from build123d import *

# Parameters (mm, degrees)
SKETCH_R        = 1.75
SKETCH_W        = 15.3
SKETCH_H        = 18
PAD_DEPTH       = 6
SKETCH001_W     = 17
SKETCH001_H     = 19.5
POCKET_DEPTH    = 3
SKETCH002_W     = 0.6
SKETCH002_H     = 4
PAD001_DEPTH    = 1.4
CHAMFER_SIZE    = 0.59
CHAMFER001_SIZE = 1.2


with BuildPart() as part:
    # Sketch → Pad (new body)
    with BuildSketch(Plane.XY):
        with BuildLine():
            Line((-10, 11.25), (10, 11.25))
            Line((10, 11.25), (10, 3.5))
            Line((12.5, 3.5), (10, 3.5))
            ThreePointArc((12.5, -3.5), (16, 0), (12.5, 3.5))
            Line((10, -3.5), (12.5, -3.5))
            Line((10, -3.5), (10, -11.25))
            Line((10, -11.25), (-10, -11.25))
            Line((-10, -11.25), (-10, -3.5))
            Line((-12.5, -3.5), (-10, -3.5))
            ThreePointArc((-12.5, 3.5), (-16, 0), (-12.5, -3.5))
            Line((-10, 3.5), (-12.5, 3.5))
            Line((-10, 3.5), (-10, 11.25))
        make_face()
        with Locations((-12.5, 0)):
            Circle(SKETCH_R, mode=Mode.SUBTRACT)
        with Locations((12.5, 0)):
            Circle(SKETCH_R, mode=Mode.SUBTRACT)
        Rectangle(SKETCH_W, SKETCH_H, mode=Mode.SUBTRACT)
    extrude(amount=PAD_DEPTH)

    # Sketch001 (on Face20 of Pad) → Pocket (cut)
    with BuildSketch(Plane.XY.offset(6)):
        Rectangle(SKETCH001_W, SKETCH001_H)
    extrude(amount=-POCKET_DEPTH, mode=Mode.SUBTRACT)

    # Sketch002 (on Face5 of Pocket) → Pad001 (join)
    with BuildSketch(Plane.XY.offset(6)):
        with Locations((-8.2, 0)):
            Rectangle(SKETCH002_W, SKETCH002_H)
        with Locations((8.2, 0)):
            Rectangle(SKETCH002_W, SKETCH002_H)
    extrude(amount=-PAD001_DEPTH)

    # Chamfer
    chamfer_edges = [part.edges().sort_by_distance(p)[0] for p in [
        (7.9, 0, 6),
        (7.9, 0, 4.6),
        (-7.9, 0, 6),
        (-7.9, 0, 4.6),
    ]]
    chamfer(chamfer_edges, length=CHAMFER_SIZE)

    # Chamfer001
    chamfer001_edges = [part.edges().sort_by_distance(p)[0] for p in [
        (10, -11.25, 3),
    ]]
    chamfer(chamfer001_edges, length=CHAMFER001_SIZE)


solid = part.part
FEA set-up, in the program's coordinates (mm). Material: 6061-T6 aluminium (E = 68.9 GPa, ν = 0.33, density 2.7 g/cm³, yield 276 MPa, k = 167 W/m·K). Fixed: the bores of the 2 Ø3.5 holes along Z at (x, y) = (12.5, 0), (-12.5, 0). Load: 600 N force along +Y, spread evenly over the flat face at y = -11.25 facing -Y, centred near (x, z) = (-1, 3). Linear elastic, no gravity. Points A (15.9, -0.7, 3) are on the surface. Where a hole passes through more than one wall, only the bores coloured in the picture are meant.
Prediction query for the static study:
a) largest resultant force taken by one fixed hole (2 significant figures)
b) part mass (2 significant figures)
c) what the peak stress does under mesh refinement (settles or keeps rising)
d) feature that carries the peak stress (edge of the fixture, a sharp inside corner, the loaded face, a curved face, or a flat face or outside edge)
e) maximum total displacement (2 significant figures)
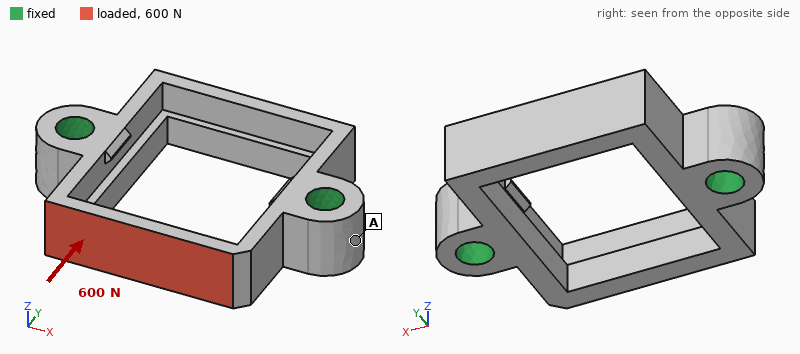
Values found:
350 N
3.3 g
keeps rising
a sharp inside corner
72 µm
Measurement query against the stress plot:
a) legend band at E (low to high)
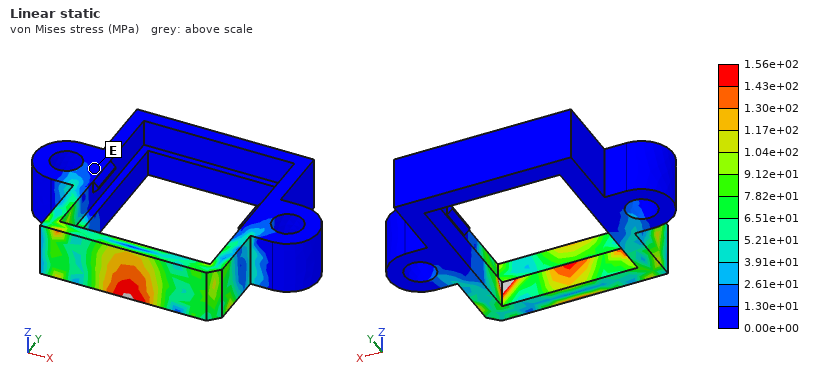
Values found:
0.00e+00 to 1.30e+01 MPa
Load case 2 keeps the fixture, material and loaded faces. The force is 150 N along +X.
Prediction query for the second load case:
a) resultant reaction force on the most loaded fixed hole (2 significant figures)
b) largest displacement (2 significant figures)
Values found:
83 N
22 µm
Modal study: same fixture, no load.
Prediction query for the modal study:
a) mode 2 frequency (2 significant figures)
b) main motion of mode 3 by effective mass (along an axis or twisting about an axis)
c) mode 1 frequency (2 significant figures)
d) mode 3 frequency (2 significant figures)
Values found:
17 kHz
twisting about X
16 kHz
19 kHz
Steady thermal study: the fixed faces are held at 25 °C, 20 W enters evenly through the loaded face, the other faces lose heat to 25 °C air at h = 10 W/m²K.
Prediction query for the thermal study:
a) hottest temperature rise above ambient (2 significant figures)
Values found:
65 K
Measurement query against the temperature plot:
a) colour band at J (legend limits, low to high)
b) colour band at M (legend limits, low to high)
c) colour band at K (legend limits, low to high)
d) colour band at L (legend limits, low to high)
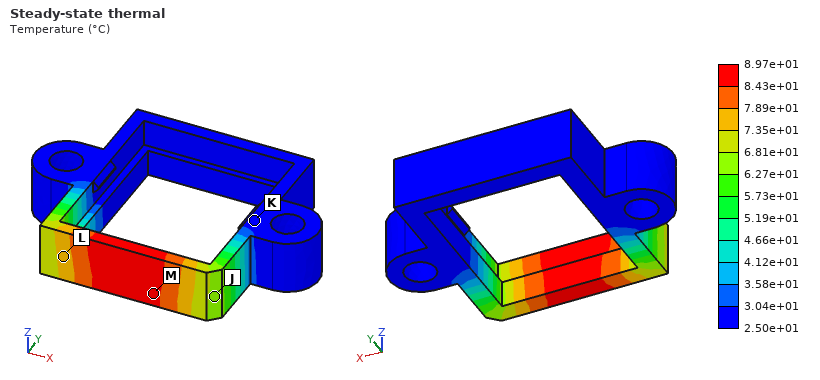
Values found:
6.27e+01 to 6.81e+01 °C
8.43e+01 to 8.97e+01 °C
2.50e+01 to 3.04e+01 °C
7.35e+01 to 7.89e+01 °C
